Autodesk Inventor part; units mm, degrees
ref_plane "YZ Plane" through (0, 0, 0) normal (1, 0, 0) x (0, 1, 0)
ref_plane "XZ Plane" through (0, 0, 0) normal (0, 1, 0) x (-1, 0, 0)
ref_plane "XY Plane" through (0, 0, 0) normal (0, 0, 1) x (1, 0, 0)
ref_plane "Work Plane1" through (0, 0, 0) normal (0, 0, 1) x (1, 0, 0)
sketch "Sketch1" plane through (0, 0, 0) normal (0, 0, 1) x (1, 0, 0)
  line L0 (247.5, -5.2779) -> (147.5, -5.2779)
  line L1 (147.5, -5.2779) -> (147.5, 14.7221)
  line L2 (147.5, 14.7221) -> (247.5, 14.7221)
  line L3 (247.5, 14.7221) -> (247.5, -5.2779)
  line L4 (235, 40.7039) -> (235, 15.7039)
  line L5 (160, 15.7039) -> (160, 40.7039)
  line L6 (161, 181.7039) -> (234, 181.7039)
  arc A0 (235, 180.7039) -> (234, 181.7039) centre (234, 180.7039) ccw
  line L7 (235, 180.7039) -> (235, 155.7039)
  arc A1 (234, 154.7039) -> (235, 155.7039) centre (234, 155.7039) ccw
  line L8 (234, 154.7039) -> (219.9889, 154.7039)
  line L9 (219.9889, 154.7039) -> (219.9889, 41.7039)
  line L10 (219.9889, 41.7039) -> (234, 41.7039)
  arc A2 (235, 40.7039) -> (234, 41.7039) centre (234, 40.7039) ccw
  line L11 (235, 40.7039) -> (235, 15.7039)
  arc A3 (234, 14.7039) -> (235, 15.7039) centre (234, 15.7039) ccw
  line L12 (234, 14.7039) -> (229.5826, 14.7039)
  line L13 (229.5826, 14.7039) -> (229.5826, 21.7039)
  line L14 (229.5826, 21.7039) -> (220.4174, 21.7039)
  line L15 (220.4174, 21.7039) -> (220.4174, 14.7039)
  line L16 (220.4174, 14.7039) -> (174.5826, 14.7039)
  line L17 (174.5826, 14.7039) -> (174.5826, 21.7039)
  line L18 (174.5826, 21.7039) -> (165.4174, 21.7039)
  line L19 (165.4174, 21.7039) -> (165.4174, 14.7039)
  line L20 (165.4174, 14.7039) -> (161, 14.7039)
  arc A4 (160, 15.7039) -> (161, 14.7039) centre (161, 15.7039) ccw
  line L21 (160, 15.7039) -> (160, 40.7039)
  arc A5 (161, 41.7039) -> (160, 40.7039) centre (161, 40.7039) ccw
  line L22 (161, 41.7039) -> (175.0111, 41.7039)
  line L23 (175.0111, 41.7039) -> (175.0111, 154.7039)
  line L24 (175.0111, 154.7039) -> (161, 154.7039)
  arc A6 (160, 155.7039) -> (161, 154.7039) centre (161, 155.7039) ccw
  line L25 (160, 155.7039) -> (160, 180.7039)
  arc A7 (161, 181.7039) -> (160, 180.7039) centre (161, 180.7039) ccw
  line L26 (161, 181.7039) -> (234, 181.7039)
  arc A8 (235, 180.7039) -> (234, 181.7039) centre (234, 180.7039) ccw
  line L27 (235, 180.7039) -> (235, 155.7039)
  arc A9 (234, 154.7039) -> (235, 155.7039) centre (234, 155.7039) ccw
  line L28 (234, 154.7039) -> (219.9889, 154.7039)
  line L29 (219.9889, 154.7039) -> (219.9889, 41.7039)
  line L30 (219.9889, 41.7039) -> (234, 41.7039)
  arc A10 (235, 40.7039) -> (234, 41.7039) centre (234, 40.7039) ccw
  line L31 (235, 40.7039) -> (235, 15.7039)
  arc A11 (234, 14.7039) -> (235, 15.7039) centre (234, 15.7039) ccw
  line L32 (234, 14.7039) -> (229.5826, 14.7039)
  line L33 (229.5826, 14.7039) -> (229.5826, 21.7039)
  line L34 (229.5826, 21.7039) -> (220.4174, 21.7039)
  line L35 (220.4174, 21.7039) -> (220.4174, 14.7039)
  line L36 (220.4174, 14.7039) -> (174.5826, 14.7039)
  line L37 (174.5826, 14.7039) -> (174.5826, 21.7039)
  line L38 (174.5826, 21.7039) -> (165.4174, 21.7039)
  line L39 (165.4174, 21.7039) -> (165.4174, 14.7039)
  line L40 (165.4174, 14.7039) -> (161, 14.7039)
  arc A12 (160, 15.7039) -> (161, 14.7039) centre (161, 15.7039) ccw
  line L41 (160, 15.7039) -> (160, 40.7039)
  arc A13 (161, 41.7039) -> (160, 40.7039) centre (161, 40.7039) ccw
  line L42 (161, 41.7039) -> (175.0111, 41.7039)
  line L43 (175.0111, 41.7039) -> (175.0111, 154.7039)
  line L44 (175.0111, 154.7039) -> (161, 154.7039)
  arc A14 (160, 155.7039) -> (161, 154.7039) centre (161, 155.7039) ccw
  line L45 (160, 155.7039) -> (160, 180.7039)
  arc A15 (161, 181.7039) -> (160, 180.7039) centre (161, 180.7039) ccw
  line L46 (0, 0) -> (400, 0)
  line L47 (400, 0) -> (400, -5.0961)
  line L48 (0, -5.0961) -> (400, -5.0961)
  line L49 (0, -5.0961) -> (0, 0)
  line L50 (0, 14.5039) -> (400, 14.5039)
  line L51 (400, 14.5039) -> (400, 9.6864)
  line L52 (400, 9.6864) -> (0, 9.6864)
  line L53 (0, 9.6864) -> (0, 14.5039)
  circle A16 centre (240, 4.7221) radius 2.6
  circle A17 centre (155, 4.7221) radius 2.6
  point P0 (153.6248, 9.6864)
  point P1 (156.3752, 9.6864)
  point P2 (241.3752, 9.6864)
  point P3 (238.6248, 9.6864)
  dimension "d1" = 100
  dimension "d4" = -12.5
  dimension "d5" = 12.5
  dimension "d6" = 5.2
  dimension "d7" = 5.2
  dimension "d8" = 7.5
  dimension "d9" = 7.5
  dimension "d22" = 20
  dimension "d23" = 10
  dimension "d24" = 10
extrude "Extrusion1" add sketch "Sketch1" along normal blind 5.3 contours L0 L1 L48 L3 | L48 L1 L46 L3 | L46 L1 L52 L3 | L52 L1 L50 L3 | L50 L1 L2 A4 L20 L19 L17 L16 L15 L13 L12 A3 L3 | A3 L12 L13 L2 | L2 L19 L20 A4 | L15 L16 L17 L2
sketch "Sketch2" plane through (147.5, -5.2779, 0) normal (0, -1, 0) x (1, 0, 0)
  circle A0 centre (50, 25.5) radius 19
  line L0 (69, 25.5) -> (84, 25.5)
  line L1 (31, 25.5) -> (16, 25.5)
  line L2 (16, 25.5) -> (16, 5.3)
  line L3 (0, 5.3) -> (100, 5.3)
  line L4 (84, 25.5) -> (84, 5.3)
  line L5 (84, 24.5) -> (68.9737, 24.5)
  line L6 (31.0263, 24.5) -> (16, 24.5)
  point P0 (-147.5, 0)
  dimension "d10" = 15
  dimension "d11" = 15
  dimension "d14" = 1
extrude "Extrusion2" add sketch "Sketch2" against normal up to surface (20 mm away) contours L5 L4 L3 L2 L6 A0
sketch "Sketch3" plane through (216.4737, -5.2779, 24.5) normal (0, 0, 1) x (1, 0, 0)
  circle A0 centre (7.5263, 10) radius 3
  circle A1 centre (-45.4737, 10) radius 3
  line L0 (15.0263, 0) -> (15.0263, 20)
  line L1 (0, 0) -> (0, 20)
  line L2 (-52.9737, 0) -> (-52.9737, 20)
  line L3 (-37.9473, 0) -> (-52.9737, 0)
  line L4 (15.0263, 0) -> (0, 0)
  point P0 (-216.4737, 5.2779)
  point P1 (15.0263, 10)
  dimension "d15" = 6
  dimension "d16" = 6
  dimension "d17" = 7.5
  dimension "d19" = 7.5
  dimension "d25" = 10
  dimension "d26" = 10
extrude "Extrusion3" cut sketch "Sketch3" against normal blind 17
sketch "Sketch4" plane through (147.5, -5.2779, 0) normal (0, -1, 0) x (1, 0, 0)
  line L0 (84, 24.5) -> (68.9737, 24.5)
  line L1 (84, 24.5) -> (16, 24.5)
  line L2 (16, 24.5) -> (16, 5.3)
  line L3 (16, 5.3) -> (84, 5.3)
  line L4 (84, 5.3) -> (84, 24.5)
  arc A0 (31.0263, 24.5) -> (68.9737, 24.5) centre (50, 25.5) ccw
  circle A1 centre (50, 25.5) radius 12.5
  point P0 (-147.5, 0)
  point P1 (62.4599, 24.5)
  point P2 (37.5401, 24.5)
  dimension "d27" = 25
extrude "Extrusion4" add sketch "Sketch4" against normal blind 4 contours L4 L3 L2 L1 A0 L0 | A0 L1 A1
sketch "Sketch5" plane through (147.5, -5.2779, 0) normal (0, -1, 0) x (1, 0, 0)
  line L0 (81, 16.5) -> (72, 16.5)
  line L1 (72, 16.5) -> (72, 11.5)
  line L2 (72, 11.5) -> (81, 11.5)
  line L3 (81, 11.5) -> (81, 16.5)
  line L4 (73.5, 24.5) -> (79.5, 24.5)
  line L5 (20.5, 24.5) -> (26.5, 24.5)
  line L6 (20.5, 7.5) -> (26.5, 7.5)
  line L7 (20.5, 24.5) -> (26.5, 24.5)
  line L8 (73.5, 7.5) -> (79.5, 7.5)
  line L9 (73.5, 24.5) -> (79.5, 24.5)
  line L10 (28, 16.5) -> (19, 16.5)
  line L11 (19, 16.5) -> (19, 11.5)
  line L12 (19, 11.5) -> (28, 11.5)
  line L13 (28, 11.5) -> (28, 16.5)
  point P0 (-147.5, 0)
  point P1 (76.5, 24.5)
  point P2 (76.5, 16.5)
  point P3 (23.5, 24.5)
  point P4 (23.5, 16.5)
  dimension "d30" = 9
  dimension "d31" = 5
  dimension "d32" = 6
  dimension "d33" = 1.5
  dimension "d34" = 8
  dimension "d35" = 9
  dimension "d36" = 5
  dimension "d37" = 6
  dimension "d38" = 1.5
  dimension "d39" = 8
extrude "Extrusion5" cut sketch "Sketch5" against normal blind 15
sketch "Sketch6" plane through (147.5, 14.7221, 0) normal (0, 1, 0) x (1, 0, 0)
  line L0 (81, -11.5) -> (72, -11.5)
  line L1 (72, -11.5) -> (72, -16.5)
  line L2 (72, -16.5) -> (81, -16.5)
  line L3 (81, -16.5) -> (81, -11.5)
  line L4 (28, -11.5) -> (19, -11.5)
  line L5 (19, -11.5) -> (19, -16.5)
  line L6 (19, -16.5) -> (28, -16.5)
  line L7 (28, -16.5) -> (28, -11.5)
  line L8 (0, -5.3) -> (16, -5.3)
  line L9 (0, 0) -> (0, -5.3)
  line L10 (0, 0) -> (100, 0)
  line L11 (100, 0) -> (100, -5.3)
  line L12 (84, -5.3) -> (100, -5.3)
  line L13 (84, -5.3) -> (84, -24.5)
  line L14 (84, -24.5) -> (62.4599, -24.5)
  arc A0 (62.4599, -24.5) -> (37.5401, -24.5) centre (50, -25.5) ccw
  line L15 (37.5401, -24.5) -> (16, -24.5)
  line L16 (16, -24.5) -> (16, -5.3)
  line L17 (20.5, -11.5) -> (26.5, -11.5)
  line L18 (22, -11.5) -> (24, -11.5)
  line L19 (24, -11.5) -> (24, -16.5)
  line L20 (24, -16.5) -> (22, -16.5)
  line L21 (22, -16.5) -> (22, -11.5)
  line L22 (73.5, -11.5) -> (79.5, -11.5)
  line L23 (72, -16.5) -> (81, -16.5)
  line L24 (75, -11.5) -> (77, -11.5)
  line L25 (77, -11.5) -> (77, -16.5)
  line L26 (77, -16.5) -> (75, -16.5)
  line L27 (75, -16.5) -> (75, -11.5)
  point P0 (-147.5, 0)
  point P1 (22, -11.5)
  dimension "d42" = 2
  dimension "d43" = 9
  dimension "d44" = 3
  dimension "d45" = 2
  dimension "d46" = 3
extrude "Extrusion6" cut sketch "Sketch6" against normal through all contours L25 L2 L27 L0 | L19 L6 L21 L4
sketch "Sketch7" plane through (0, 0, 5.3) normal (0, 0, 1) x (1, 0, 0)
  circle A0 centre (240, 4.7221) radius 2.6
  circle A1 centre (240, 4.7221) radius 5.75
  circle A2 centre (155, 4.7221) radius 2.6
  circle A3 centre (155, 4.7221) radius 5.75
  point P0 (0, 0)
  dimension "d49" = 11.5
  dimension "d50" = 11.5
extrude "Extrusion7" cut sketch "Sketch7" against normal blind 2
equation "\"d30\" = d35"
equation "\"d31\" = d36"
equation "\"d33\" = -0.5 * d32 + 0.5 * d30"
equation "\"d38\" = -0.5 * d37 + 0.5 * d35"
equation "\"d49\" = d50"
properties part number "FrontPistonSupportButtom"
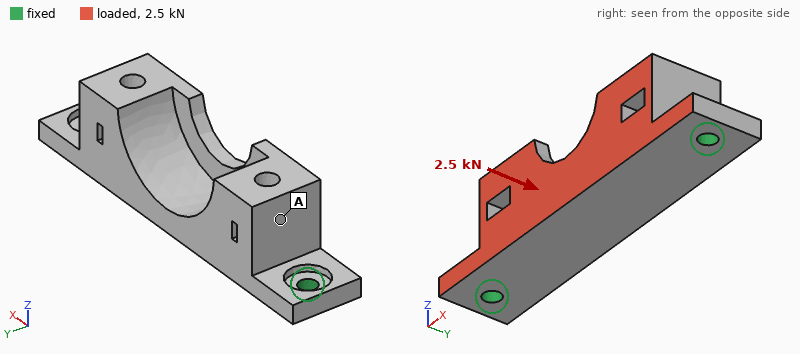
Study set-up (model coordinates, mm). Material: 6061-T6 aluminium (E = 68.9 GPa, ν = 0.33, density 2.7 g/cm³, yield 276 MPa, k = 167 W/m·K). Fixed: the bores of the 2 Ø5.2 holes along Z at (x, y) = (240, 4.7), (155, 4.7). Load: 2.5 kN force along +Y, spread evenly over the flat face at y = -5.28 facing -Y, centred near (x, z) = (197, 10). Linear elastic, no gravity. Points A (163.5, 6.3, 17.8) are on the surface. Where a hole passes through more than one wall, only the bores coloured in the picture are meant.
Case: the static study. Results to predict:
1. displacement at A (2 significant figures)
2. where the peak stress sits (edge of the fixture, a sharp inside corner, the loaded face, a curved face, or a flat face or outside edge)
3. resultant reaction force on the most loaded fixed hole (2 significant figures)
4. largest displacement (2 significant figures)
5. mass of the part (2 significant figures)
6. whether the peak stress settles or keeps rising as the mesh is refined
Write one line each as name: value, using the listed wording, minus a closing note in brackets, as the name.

displacement at A: 0.11 mm
where the peak stress sits: edge of the fixture
resultant reaction force on the most loaded fixed hole: 1.3 kN
largest displacement: 0.18 mm
mass of the part: 67 g
whether the peak stress settles or keeps rising as the mesh is refined: keeps rising
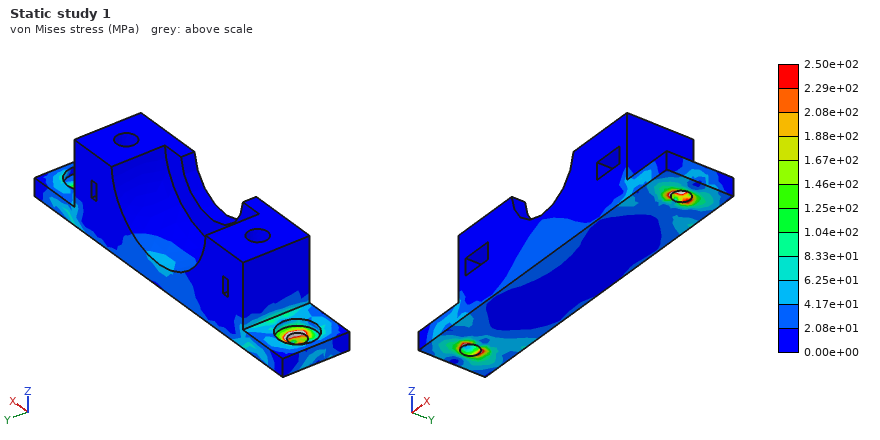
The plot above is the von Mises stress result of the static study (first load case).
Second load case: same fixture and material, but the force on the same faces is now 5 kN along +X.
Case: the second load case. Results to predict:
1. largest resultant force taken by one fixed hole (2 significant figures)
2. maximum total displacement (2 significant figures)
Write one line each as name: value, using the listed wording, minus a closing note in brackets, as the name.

largest resultant force taken by one fixed hole: 2.6 kN
maximum total displacement: 19 µm
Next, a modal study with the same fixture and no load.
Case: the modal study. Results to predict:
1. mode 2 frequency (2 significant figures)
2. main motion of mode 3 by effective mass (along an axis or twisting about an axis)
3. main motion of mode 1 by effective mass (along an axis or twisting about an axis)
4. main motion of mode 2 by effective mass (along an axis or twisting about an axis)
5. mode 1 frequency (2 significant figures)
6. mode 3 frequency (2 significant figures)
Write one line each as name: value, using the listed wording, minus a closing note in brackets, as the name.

mode 2 frequency: 4000 Hz
main motion of mode 3 by effective mass: twisting about Z
main motion of mode 1 by effective mass: along Y
main motion of mode 2 by effective mass: along Z
mode 1 frequency: 2900 Hz
mode 3 frequency: 6500 Hz
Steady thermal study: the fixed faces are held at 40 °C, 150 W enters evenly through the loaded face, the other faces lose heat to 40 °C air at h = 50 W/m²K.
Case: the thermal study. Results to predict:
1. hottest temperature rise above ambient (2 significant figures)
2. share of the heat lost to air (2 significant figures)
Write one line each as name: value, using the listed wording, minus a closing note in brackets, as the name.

hottest temperature rise above ambient: 73 K
share of the heat lost to air: 14 %
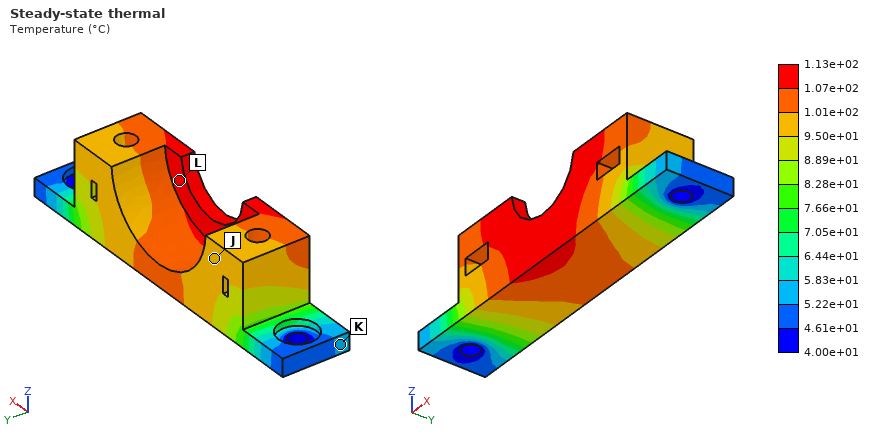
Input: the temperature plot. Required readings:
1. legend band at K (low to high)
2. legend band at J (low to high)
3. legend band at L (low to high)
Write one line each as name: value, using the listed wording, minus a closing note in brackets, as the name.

legend band at K: 5.22e+01 to 5.83e+01 °C
legend band at J: 9.50e+01 to 1.01e+02 °C
legend band at L: 1.07e+02 to 1.13e+02 °C
